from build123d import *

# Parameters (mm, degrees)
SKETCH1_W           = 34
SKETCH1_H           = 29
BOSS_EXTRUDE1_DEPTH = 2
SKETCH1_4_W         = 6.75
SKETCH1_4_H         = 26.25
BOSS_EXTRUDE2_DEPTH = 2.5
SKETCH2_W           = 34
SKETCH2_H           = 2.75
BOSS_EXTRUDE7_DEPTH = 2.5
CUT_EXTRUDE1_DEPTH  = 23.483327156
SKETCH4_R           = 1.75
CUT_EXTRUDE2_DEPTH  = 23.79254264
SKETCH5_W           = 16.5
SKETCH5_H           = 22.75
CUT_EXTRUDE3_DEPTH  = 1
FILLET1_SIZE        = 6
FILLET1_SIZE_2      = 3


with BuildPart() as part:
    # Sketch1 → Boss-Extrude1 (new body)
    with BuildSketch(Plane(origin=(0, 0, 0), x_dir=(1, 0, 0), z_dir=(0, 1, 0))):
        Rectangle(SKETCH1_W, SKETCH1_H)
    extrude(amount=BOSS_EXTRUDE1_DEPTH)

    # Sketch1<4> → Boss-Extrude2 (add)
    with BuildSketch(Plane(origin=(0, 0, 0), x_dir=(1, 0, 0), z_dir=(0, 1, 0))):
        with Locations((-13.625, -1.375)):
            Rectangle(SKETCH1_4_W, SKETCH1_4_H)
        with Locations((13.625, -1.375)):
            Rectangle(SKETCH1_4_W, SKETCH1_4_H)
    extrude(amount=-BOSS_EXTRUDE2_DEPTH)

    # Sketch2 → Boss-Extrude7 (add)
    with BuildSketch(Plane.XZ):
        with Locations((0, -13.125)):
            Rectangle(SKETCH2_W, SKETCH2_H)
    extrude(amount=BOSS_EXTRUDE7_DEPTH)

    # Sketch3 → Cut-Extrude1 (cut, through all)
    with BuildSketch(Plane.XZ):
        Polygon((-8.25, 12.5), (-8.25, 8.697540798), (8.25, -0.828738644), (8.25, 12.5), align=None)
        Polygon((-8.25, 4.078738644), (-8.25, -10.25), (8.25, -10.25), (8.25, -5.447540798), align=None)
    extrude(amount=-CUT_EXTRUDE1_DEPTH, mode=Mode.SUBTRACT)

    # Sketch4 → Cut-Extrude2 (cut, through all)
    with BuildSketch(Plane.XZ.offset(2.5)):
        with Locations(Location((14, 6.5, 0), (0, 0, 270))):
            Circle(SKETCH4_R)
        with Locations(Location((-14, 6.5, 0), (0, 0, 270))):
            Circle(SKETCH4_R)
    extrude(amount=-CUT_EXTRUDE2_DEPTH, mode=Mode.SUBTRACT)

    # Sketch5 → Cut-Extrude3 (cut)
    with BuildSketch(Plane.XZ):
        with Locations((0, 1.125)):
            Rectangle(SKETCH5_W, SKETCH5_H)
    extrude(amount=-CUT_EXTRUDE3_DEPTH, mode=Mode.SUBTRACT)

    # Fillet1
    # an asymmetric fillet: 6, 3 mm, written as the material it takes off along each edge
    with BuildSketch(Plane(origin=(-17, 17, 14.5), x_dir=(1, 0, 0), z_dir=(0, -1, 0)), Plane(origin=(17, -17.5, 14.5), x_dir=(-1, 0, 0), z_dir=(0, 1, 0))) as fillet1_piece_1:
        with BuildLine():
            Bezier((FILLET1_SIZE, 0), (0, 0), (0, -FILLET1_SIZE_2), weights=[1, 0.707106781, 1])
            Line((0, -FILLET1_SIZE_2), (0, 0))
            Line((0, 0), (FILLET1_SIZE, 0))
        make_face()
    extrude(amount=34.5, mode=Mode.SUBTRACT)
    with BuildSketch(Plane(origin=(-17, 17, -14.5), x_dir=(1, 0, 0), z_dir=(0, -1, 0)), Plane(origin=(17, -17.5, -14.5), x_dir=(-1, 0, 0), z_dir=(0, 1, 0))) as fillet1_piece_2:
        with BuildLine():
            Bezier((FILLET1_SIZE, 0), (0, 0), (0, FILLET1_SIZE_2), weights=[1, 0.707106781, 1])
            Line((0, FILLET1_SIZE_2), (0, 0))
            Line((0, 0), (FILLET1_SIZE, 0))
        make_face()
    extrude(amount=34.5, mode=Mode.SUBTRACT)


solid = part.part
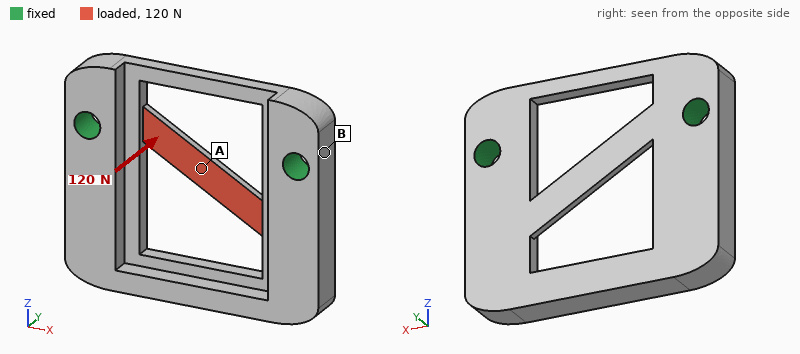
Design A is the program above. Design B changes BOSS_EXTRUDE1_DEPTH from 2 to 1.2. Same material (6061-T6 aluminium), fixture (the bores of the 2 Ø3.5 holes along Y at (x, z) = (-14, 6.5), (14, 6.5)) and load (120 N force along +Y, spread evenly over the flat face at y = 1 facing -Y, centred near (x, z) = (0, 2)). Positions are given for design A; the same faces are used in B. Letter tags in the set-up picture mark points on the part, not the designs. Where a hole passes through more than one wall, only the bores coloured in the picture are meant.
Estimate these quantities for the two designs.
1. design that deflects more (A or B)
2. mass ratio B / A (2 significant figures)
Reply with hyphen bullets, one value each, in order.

- B
- 0.77
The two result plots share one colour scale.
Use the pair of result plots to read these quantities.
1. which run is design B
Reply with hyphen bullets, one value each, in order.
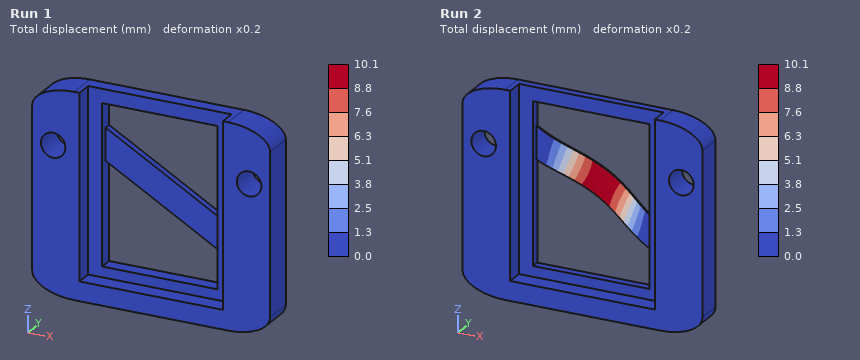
- Run 2
